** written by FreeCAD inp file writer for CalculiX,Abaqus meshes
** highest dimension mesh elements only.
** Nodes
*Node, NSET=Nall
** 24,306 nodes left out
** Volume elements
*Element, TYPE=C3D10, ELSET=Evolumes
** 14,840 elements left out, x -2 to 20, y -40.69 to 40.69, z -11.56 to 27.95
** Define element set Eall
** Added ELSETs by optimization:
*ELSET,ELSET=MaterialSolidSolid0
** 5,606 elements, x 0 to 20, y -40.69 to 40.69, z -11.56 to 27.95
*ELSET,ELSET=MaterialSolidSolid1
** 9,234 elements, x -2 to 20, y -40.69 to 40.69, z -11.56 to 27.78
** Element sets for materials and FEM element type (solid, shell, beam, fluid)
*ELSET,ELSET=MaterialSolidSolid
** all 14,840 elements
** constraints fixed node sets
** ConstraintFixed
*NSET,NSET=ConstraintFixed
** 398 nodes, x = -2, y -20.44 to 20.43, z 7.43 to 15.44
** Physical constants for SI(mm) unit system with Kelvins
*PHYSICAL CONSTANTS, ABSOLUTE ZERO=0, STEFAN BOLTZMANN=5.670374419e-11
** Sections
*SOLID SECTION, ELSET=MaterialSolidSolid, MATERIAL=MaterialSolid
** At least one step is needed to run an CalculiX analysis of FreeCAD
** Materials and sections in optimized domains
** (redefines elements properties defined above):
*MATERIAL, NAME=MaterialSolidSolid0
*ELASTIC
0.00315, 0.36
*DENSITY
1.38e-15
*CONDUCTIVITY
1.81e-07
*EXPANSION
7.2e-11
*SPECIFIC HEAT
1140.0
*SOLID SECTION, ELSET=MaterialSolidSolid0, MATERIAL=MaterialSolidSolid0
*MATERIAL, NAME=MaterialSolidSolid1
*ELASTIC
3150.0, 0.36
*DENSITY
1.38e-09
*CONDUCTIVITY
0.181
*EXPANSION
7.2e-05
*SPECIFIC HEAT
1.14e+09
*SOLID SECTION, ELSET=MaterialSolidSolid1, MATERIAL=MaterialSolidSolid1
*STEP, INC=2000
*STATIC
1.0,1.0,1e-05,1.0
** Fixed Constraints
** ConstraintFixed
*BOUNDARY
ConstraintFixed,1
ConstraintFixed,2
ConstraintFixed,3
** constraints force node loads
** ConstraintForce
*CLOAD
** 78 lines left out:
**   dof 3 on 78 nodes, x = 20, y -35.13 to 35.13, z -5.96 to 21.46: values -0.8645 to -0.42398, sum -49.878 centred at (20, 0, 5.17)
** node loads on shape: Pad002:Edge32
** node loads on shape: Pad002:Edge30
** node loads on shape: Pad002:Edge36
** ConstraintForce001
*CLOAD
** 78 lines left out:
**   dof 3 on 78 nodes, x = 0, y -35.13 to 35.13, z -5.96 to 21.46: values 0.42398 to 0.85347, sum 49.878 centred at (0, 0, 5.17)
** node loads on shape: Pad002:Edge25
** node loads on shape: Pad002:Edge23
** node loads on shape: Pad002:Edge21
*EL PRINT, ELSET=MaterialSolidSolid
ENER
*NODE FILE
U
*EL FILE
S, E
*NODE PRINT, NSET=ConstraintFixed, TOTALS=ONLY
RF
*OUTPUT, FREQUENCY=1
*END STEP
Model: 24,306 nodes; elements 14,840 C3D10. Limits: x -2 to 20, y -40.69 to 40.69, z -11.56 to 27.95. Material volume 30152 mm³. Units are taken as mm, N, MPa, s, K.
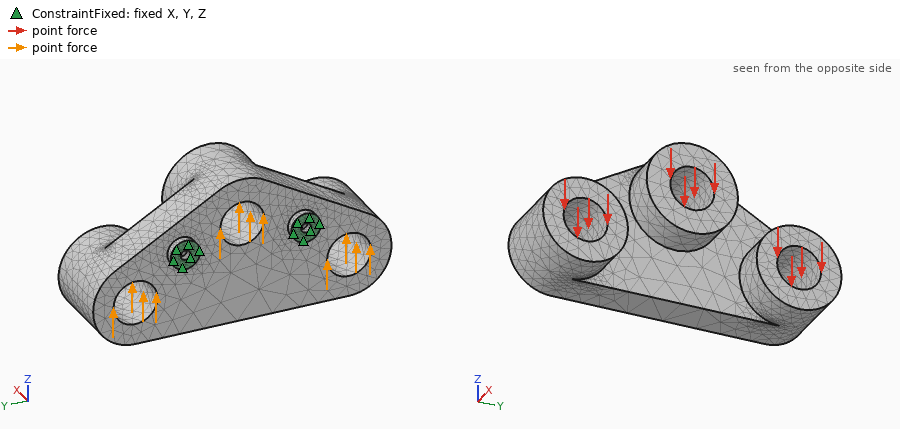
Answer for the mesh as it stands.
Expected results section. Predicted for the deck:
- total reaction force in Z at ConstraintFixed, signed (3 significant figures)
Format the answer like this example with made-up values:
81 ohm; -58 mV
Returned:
-3.16e-06 N
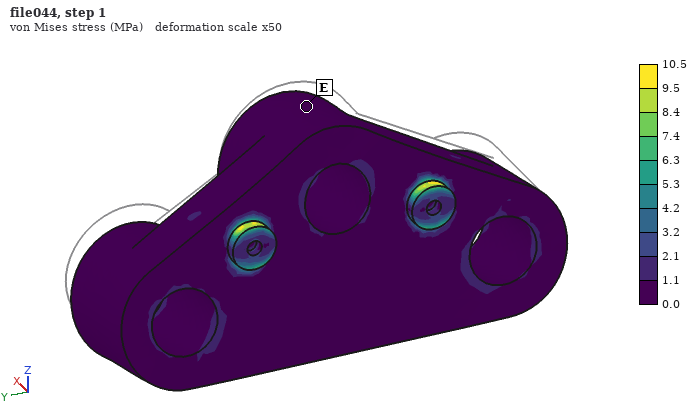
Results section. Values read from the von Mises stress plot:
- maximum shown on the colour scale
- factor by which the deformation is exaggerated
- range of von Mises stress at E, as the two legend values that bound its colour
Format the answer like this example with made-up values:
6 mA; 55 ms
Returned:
10.5 MPa; 50; 0.0 to 1.1 MPa
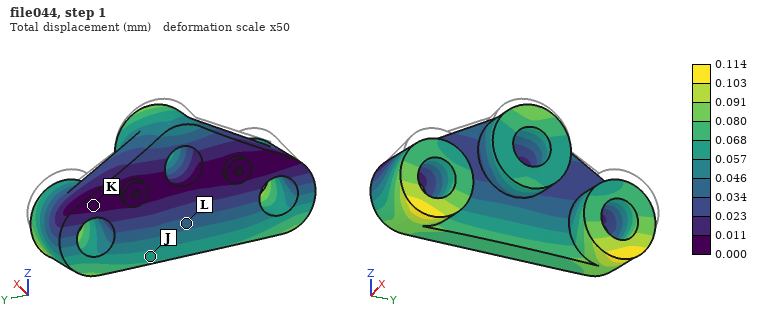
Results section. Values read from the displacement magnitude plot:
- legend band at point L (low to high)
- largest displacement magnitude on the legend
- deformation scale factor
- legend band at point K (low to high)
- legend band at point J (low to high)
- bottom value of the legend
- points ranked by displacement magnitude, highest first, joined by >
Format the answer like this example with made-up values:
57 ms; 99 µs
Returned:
0.034 to 0.046 mm; 0.114 mm; 50; 0.000 to 0.011 mm; 0.057 to 0.068 mm; 0.000 mm; J > L > K
